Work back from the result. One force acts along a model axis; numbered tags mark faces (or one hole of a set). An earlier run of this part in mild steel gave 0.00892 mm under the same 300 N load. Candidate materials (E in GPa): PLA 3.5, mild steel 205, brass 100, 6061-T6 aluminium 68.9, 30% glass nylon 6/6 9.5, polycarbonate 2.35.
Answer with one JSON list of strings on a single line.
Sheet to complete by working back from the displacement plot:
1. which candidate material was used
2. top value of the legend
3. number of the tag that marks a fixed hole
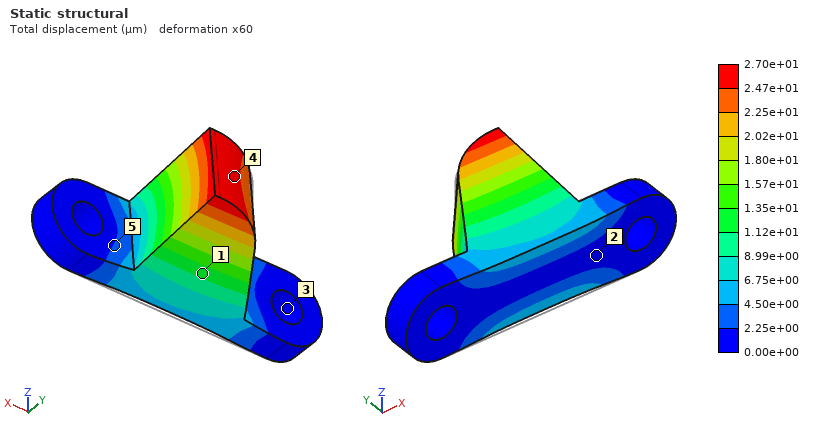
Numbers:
["6061-T6 aluminium", "2.70e+01 µm", "3"]
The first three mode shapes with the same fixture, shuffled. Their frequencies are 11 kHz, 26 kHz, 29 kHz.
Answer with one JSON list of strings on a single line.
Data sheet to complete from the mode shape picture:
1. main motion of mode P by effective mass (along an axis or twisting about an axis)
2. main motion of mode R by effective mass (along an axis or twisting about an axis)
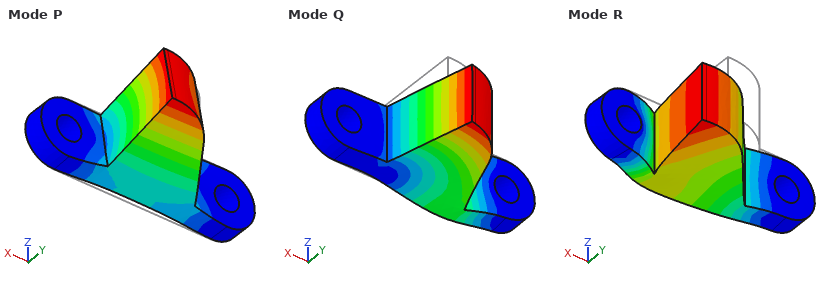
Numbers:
["along Z", "along Y"]
